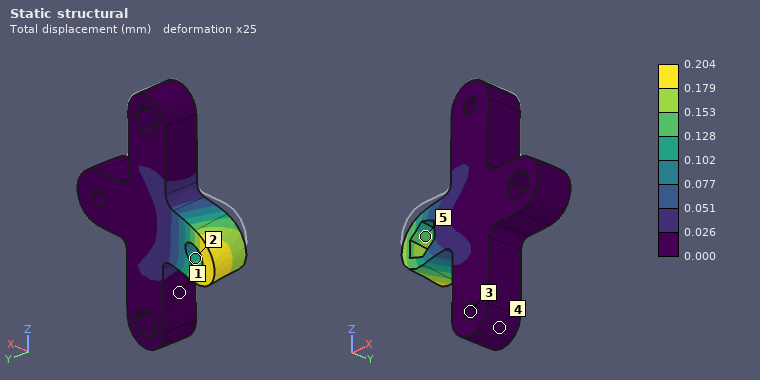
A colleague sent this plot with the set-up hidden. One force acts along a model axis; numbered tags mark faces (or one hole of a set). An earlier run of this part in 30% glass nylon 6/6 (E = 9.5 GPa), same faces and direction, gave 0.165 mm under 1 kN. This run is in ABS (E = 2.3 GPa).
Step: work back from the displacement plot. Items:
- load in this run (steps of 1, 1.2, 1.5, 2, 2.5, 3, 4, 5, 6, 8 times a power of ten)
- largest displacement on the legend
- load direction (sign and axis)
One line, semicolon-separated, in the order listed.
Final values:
300 N; 0.204 mm; -Z
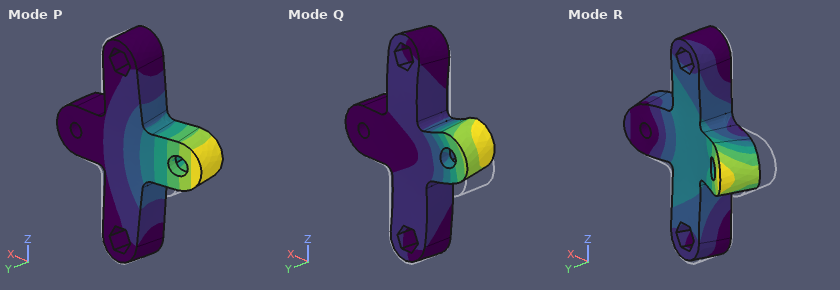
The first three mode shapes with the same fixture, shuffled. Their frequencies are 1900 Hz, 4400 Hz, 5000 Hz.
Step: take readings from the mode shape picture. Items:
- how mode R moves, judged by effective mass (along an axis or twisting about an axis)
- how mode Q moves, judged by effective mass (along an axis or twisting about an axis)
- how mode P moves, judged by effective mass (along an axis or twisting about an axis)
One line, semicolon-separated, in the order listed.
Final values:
along X; along Z; along Y
